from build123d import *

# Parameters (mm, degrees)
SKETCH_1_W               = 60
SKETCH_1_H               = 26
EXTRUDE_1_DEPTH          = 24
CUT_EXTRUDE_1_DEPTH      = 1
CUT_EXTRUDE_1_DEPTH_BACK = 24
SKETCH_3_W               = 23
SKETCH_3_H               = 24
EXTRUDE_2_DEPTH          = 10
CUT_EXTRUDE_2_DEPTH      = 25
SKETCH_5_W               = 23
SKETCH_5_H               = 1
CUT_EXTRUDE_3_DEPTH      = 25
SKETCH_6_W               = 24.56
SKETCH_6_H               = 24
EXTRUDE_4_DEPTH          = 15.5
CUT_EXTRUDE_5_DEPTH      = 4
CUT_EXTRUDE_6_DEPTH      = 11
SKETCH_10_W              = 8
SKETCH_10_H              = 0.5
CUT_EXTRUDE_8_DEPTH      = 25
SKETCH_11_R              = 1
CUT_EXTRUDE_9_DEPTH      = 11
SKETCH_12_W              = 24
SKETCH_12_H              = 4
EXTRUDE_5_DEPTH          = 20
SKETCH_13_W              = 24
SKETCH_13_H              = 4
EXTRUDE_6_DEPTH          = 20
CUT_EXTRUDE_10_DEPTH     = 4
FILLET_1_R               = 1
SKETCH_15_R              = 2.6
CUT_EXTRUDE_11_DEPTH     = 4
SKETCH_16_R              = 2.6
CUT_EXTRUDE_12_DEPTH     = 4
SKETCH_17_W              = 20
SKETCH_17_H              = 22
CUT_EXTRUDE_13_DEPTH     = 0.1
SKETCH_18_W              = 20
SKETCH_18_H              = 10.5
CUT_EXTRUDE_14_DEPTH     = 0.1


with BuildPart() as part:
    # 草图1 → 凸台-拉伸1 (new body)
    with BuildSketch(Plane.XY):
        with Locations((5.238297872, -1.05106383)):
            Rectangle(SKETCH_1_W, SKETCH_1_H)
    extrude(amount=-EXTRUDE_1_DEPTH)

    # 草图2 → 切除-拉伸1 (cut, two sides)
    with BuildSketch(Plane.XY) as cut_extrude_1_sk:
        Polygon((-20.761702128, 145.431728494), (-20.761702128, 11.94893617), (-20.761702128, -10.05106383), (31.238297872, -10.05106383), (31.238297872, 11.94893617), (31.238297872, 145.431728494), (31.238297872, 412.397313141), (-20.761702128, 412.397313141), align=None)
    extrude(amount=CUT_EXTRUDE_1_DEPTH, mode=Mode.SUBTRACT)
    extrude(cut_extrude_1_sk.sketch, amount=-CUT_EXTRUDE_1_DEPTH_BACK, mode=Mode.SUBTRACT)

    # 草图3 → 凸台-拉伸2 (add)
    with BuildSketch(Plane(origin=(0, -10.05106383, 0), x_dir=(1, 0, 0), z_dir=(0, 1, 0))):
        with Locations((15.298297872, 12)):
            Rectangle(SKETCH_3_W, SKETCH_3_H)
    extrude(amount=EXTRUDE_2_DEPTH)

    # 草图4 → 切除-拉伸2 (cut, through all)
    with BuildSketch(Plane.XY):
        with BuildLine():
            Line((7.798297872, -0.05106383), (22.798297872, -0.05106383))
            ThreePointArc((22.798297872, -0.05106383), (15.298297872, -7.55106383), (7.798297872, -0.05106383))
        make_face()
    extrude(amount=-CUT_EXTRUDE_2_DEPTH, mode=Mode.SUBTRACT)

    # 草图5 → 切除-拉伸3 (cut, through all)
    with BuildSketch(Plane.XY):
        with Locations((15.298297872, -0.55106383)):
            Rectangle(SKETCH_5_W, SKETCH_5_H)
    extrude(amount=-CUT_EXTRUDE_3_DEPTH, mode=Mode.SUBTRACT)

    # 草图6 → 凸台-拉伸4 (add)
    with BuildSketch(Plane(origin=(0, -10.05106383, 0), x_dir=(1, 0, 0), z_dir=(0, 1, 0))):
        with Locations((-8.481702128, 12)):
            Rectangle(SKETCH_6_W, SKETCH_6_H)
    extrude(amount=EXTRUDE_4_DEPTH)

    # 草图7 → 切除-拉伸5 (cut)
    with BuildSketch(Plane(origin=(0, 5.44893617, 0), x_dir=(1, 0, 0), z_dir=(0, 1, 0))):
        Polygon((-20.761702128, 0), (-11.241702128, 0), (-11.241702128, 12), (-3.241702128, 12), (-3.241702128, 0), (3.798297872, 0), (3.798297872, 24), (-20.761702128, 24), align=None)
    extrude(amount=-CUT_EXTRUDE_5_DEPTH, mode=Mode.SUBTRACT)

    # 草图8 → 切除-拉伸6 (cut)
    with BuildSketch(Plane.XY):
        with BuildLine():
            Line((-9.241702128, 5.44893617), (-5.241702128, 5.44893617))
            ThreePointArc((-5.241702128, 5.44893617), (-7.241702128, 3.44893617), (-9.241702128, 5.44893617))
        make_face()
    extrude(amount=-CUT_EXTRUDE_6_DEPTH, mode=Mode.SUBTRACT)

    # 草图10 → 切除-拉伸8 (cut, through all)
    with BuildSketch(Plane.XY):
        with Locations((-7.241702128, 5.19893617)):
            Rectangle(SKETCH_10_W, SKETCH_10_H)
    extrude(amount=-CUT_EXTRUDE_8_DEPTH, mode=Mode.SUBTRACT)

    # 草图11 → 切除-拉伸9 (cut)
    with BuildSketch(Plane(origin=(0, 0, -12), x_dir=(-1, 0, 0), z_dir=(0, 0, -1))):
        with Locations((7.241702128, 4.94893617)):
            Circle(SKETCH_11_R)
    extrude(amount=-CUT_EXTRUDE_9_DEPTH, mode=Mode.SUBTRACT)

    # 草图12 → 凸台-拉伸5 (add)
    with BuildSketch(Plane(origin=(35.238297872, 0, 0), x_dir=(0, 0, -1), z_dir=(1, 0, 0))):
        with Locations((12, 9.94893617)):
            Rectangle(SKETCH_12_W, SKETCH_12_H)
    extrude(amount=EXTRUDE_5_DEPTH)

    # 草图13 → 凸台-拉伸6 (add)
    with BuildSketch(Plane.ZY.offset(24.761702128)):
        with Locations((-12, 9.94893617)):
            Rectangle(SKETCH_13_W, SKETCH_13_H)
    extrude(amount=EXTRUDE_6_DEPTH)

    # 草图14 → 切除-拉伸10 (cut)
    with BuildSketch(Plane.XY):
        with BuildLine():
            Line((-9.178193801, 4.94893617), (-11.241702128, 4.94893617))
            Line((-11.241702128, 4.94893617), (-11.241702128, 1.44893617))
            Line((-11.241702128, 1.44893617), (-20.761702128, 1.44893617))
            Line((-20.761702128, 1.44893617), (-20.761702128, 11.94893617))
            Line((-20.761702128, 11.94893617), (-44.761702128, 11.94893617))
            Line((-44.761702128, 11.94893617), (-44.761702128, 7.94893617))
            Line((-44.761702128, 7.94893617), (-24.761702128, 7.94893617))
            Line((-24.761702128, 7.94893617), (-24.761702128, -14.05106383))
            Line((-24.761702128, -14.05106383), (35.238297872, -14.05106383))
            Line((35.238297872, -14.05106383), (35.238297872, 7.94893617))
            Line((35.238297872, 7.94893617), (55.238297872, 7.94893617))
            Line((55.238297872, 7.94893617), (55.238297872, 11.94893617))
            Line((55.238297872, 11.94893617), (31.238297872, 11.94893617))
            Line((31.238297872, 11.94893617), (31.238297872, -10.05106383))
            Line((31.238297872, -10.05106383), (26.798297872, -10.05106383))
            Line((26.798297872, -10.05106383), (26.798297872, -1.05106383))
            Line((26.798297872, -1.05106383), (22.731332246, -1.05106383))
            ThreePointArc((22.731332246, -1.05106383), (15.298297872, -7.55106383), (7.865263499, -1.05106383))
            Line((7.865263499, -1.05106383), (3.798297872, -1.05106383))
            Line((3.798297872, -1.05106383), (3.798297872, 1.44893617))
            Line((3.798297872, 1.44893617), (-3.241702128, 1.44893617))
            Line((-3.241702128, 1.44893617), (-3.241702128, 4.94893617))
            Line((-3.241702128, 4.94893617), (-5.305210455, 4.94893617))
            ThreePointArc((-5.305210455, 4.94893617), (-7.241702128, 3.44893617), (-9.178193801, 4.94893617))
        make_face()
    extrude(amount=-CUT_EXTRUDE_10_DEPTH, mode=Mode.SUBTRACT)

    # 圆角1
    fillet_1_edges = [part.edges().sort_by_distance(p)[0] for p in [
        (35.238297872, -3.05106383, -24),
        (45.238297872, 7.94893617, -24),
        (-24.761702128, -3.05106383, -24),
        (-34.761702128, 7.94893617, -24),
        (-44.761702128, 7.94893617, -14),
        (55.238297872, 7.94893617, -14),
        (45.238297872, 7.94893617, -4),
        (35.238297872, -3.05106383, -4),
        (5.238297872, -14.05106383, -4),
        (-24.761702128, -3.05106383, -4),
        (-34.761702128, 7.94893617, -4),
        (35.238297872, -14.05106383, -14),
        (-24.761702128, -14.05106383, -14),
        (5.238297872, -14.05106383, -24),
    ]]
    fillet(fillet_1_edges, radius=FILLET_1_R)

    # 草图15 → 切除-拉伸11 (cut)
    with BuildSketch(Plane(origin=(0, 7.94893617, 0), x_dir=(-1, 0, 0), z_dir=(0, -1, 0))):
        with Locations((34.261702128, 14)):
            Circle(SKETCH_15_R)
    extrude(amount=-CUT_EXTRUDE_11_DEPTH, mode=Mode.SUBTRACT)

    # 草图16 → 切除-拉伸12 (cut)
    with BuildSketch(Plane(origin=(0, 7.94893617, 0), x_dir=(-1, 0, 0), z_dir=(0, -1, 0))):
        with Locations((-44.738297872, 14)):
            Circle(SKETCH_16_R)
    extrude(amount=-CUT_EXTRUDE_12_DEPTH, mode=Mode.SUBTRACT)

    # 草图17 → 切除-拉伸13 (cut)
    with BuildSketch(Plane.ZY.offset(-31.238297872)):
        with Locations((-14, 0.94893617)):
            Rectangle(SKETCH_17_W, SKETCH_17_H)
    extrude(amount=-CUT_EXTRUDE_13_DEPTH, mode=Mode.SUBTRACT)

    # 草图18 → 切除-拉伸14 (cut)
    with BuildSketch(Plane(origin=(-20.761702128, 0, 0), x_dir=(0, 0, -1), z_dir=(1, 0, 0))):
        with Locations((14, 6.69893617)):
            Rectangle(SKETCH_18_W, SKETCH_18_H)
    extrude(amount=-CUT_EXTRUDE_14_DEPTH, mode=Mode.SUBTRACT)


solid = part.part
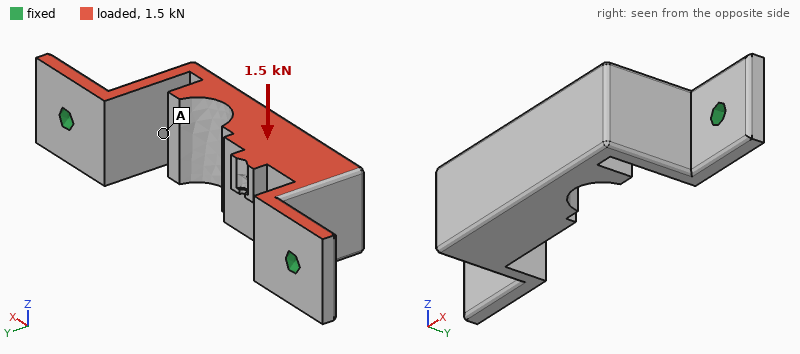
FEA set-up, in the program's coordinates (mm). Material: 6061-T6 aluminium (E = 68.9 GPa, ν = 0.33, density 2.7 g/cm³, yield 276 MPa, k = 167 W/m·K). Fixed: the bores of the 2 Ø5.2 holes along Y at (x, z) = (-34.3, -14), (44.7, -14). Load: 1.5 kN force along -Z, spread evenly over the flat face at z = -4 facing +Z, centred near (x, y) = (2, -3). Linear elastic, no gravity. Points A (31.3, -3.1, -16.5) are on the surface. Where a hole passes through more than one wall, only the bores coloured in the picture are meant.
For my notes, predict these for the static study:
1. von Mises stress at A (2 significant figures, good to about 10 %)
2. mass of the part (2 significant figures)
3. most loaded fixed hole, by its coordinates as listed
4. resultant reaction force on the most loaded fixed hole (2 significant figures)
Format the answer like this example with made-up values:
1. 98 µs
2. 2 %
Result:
1. 23 MPa
2. 53 g
3. (-34.3, -14)
4. 850 N
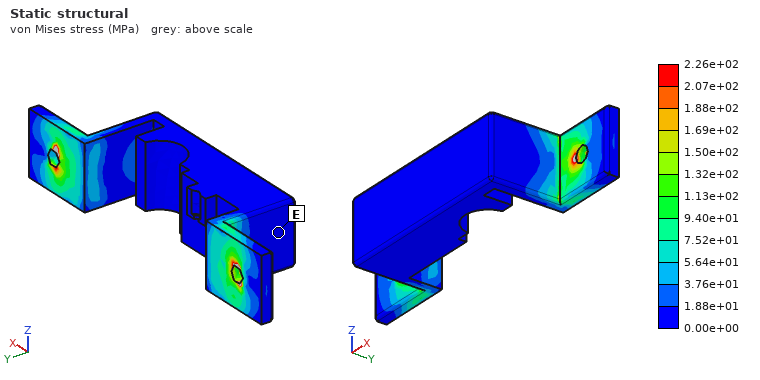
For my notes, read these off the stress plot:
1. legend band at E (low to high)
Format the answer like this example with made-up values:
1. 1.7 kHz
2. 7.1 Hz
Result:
1. 0.00e+00 to 1.88e+01 MPa
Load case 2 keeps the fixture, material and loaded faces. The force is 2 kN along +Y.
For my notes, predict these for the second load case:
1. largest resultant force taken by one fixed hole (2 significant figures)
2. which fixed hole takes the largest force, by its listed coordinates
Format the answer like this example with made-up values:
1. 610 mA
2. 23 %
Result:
1. 1.2 kN
2. (-34.3, -14)
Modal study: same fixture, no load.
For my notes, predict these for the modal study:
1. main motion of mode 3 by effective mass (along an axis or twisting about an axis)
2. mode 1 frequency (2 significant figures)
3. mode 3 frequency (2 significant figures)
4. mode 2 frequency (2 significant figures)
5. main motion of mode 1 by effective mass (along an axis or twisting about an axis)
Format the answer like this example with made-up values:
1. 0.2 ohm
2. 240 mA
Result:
1. twisting about Y
2. 2100 Hz
3. 5300 Hz
4. 3800 Hz
5. along Z
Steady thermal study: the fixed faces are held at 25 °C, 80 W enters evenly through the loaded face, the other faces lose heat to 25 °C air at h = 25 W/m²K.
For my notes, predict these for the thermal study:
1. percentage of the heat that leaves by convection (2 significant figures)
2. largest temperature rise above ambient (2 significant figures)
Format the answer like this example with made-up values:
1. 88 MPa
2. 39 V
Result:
1. 9.7 %
2. 73 K
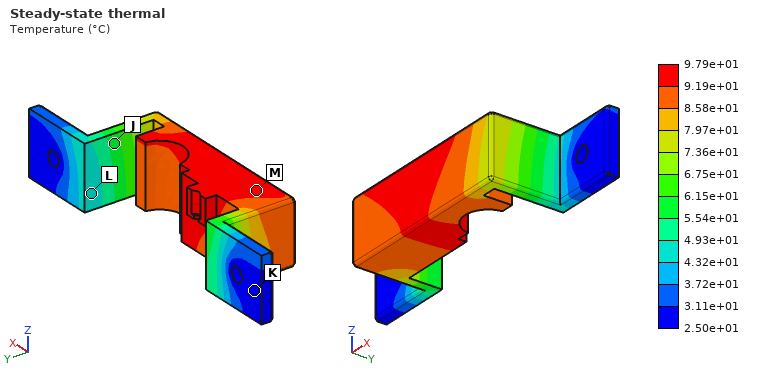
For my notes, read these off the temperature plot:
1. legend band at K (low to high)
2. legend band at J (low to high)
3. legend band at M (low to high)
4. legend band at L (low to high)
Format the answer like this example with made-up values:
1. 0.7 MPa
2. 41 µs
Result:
1. 2.50e+01 to 3.11e+01 °C
2. 5.54e+01 to 6.15e+01 °C
3. 9.19e+01 to 9.79e+01 °C
4. 4.32e+01 to 4.93e+01 °C
